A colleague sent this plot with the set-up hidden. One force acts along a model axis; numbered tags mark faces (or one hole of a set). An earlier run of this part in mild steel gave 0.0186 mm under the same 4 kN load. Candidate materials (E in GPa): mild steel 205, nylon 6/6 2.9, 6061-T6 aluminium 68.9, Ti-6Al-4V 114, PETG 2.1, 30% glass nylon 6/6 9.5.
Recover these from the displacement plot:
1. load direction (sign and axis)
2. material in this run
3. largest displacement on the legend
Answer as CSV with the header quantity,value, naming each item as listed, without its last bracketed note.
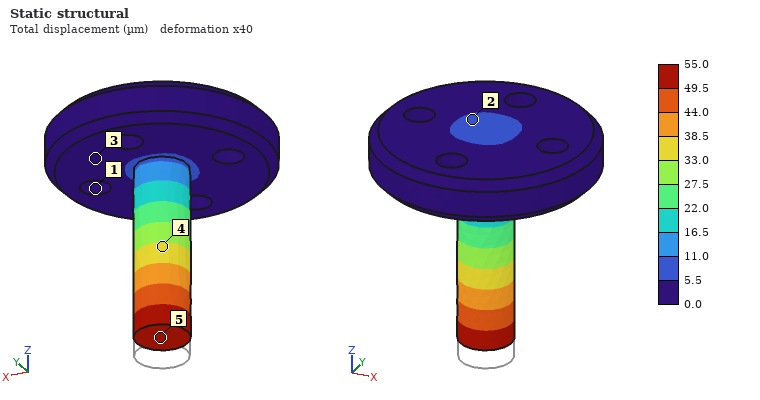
quantity,value
load direction,+Z
material in this run,6061-T6 aluminium
largest displacement on the legend,55.0 µm
